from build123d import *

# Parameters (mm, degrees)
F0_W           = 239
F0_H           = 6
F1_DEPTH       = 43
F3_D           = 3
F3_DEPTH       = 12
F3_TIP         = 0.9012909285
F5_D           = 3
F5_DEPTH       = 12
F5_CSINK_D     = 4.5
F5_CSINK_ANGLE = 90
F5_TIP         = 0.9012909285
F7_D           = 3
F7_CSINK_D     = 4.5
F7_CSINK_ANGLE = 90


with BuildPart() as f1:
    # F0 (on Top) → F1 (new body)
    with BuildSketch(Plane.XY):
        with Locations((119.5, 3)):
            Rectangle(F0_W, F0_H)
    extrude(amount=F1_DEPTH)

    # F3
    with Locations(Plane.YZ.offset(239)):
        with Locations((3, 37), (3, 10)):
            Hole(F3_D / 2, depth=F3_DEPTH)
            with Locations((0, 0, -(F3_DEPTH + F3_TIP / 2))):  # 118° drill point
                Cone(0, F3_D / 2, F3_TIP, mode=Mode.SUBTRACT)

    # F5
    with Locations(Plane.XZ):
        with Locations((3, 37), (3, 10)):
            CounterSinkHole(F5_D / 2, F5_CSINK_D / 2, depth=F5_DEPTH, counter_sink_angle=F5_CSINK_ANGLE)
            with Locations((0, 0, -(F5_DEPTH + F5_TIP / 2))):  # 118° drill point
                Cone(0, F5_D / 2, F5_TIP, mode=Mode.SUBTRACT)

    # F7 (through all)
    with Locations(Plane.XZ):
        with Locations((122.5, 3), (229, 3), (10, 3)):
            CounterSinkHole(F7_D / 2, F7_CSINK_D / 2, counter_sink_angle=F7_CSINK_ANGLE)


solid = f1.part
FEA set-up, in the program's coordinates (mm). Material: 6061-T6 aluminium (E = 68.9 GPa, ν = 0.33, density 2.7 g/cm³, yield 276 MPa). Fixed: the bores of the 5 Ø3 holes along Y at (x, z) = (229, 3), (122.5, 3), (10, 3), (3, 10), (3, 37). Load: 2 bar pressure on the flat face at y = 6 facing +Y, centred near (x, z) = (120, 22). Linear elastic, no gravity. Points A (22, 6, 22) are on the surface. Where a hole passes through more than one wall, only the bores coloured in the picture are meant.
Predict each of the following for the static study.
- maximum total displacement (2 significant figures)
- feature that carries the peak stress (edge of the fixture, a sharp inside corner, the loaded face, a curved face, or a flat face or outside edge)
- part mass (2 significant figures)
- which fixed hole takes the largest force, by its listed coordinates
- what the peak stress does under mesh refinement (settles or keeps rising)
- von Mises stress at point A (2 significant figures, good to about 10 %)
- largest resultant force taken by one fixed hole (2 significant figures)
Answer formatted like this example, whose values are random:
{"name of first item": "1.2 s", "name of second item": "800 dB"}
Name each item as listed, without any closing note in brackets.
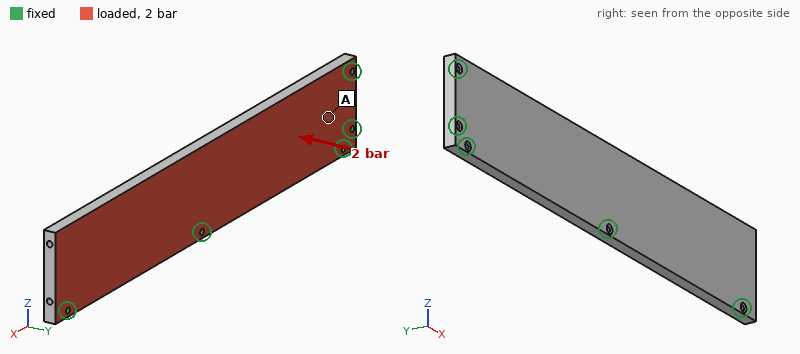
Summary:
{"maximum total displacement": "0.29 mm", "feature that carries the peak stress": "edge of the fixture", "part mass": "170 g", "which fixed hole takes the largest force, by its listed coordinates": "(122.5, 3)", "what the peak stress does under mesh refinement": "keeps rising", "von Mises stress at point A": "17 MPa", "largest resultant force taken by one fixed hole": "1000 N"}
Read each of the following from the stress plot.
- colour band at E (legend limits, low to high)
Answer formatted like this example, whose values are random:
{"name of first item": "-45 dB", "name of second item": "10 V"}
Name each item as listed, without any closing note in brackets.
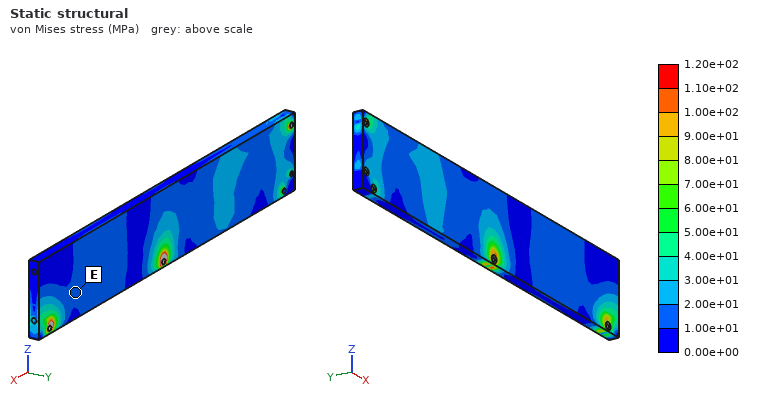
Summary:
{"colour band at E": "1.00e+01 to 2.00e+01 MPa"}
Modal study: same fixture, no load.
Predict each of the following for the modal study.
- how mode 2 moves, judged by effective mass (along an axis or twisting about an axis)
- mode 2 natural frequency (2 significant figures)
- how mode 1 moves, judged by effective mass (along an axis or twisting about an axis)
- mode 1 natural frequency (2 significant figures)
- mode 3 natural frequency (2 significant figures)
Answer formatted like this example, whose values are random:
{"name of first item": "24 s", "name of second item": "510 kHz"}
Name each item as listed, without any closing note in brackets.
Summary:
{"how mode 2 moves, judged by effective mass": "along Y", "mode 2 natural frequency": "1700 Hz", "how mode 1 moves, judged by effective mass": "along Y", "mode 1 natural frequency": "1400 Hz", "mode 3 natural frequency": "2900 Hz"}
